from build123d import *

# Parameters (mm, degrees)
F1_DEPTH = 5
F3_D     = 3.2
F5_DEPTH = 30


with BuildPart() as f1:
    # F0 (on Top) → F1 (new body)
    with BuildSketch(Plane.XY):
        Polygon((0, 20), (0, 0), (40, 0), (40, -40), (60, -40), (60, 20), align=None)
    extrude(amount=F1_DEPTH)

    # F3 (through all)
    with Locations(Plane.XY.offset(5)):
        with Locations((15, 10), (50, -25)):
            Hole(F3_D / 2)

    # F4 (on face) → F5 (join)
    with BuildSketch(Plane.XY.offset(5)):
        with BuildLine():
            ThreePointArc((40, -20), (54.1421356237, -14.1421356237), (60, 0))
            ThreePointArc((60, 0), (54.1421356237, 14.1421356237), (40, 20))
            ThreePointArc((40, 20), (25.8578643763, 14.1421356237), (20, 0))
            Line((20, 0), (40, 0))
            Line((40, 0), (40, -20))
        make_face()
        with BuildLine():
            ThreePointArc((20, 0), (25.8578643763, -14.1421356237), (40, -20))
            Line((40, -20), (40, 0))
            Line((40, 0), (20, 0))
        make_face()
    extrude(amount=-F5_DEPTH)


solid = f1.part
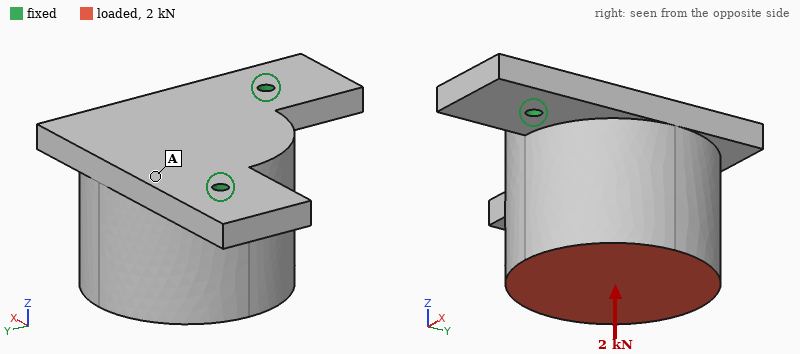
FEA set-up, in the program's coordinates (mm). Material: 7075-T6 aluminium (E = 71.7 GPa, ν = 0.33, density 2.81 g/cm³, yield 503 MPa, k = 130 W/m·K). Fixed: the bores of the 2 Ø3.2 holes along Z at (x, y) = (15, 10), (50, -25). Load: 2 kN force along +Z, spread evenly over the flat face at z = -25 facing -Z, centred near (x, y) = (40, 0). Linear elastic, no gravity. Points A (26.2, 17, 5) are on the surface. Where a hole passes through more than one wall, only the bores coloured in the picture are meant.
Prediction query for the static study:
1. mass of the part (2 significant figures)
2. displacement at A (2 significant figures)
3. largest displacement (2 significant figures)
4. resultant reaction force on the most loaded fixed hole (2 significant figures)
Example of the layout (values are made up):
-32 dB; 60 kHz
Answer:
120 g; 0.054 mm; 0.18 mm; 1.0 kN
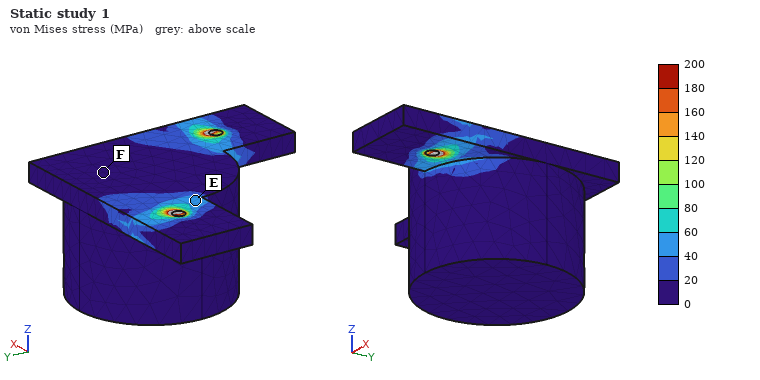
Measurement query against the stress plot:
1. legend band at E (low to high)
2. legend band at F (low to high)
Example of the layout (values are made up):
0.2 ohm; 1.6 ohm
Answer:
40 to 60 MPa; 0 to 20 MPa
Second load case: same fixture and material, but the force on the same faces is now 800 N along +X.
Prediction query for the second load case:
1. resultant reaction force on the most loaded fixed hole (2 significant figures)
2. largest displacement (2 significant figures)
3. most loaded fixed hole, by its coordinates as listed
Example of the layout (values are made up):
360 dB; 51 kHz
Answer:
750 N; 0.15 mm; (15, 10)
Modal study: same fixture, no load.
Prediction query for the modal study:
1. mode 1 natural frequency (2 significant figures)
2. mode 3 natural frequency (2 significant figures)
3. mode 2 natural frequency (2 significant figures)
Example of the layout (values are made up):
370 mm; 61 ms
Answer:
1500 Hz; 6700 Hz; 6500 Hz
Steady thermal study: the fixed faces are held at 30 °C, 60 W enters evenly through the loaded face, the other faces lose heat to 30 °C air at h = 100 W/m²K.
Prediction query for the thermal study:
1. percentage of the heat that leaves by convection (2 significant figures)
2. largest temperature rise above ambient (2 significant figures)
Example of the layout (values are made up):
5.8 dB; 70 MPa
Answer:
25 %; 33 K
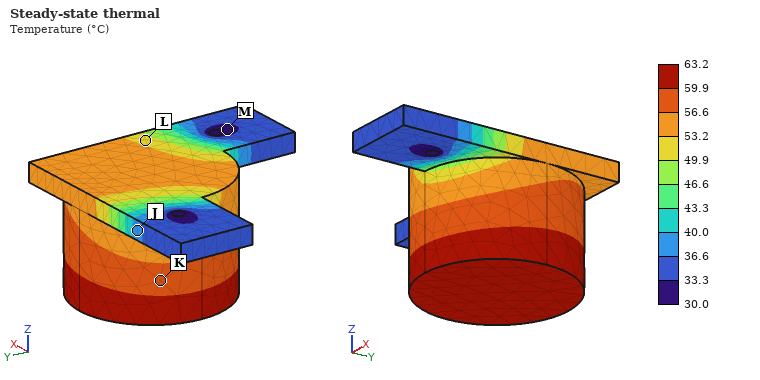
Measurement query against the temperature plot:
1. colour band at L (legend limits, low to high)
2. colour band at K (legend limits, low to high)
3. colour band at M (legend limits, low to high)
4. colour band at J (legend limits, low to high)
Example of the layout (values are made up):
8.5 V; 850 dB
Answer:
49.9 to 53.2 °C; 56.6 to 59.9 °C; 30.0 to 33.3 °C; 36.6 to 40.0 °C
